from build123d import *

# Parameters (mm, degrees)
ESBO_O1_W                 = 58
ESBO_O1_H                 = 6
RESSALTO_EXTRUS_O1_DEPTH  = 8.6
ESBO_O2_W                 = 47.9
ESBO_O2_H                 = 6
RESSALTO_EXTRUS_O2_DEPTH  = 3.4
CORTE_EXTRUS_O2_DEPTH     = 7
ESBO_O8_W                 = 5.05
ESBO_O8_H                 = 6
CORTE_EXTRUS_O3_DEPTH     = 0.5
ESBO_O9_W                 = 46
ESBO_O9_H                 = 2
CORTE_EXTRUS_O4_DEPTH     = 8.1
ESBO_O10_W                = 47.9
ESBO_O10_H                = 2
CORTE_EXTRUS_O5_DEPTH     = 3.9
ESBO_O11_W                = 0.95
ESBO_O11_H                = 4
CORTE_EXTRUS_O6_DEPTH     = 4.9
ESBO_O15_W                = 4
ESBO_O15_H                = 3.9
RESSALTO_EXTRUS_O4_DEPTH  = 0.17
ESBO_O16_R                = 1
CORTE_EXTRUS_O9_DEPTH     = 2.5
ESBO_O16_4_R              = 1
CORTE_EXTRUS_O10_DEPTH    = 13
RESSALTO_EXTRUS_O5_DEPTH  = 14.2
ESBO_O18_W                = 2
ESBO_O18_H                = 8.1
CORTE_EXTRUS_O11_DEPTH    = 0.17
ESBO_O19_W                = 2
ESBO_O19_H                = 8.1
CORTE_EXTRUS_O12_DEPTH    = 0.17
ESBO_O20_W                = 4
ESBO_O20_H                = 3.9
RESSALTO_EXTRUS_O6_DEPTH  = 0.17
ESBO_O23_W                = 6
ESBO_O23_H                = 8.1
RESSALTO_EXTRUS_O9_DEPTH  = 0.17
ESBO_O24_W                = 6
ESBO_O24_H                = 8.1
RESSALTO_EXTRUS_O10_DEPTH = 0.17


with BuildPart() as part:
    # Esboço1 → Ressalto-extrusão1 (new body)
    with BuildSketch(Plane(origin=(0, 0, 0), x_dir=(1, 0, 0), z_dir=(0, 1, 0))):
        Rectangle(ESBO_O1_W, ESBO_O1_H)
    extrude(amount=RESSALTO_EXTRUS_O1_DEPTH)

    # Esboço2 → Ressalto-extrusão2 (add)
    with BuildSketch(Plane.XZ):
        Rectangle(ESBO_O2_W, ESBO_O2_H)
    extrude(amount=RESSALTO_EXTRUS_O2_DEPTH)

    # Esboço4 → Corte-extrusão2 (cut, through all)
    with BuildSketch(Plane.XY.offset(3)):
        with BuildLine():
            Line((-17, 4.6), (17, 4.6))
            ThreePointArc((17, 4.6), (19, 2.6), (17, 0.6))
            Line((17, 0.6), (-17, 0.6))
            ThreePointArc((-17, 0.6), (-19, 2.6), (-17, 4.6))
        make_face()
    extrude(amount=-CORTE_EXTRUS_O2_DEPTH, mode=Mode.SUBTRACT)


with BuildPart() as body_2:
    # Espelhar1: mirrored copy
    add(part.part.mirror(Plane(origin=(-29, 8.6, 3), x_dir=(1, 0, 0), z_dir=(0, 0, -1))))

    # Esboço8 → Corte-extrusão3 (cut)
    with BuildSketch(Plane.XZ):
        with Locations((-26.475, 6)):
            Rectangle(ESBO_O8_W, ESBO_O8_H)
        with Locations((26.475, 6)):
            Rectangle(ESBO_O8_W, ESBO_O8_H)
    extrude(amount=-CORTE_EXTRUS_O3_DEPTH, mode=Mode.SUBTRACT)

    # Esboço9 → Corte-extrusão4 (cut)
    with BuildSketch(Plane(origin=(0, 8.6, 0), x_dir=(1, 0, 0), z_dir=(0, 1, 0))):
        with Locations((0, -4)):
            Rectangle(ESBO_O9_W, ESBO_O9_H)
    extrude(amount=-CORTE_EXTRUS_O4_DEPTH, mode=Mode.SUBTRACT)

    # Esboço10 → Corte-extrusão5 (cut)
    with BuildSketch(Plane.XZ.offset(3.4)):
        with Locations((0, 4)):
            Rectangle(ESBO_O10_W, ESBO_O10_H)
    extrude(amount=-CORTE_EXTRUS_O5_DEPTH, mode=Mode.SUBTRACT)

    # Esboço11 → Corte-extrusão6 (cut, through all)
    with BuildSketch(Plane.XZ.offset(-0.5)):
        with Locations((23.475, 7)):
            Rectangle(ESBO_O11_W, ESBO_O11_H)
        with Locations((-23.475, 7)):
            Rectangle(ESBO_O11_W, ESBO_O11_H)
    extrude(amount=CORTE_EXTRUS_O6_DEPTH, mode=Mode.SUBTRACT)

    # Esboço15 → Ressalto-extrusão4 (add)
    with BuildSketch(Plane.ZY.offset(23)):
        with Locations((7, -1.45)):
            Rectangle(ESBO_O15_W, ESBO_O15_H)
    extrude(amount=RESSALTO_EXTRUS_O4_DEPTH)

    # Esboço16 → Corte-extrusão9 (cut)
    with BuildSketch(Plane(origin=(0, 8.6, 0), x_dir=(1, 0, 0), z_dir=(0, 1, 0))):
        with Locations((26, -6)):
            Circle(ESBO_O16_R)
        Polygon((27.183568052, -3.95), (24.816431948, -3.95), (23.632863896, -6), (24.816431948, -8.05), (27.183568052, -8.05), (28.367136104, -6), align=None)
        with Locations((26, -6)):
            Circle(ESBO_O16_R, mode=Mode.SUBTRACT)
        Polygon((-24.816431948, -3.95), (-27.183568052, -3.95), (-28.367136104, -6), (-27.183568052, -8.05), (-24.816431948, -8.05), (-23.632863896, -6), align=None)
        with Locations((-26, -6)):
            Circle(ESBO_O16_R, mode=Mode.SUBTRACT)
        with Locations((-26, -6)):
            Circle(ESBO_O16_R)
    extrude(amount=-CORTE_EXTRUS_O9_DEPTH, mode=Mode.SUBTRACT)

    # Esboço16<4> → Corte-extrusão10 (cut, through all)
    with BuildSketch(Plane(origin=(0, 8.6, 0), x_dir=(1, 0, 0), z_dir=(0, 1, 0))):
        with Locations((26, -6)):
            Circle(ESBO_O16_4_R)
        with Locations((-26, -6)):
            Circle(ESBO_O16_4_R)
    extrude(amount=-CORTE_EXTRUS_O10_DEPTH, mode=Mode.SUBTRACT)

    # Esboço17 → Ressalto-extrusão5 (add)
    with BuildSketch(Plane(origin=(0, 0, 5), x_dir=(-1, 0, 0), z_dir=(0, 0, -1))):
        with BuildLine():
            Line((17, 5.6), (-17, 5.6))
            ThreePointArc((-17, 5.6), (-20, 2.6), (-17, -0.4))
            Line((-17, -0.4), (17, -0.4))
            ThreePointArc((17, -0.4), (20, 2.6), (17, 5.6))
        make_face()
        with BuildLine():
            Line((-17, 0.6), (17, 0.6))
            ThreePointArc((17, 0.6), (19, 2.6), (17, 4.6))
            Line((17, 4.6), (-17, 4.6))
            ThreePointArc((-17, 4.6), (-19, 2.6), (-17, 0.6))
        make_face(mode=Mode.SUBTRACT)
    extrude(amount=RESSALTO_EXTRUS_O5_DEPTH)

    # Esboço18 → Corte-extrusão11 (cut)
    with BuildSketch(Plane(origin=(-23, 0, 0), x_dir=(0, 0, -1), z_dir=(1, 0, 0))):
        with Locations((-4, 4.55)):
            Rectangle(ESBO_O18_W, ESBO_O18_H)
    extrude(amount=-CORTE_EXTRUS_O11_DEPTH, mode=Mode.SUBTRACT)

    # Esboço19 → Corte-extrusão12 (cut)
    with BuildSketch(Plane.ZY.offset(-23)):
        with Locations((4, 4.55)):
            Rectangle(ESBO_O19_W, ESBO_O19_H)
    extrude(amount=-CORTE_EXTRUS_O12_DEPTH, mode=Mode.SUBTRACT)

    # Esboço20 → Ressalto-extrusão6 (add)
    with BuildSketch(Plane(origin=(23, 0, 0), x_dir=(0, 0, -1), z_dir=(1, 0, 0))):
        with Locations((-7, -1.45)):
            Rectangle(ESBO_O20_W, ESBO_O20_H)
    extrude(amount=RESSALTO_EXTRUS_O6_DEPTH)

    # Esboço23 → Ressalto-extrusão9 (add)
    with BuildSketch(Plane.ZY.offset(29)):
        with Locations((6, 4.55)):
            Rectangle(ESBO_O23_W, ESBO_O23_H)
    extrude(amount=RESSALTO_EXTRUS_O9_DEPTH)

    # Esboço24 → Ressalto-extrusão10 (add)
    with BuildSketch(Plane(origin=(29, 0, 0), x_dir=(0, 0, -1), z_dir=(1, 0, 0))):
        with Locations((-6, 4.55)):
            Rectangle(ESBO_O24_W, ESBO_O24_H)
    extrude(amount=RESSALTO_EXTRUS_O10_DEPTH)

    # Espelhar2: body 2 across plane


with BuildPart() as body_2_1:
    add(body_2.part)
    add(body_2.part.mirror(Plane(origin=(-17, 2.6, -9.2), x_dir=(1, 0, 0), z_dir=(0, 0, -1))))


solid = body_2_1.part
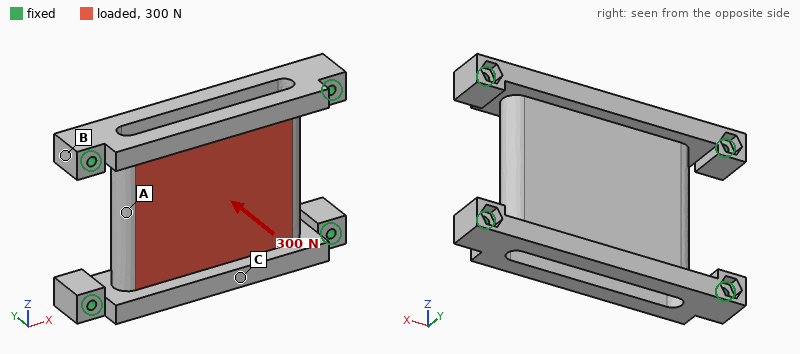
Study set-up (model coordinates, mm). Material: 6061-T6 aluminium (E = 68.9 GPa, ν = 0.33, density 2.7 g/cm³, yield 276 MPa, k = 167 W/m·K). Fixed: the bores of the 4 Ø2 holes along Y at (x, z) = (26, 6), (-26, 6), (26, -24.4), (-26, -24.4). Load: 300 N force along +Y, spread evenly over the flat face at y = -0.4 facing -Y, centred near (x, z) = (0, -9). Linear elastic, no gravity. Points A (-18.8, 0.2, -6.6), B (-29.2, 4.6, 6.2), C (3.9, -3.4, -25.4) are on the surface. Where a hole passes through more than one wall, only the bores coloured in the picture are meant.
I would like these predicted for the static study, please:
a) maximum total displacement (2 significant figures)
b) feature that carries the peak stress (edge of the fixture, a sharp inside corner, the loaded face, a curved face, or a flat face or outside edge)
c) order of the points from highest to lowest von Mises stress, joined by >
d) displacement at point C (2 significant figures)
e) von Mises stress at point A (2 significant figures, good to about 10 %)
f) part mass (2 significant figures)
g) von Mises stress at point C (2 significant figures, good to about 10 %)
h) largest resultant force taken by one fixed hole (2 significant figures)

0.11 mm
a curved face
A > C > B
0.022 mm
51 MPa
18 g
26 MPa
91 N
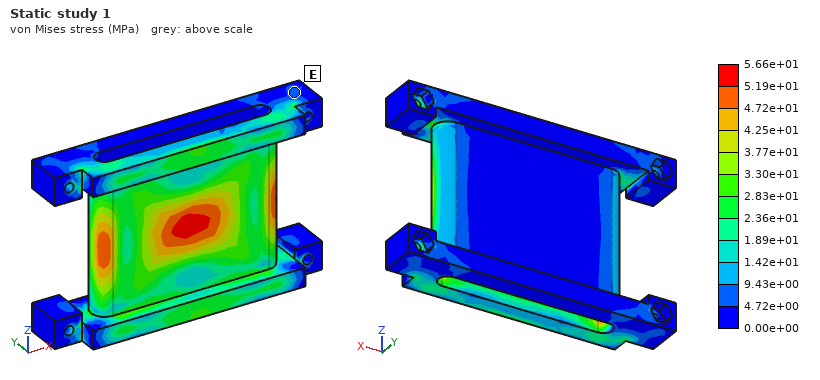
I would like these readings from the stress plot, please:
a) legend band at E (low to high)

4.72e+00 to 9.43e+00 MPa
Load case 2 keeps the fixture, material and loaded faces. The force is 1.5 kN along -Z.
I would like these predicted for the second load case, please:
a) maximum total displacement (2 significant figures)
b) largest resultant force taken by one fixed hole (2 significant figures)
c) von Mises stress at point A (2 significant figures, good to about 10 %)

30 µm
390 N
25 MPa
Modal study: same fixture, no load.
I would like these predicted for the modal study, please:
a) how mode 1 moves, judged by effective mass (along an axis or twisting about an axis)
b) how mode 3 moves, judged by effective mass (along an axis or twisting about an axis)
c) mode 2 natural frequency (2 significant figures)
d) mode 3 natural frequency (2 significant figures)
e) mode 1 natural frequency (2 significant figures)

along Y
twisting about X
6500 Hz
9300 Hz
6100 Hz
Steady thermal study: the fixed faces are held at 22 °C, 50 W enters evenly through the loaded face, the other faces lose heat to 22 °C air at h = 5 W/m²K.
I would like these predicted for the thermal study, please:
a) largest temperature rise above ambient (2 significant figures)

63 K
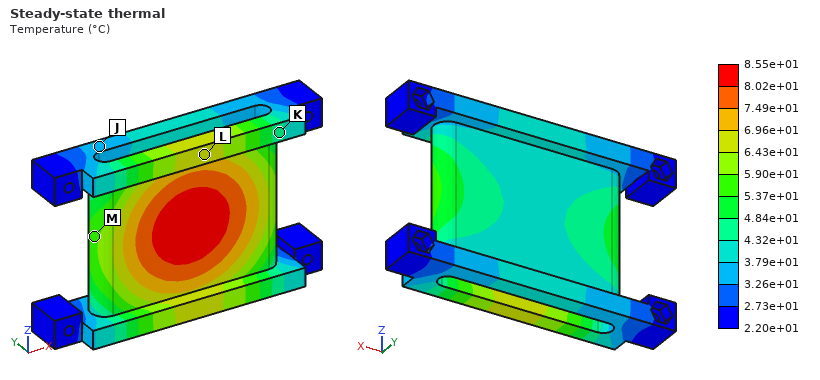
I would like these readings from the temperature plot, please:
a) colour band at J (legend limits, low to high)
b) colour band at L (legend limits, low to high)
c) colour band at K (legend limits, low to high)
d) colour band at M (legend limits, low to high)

3.26e+01 to 3.79e+01 °C
6.43e+01 to 6.96e+01 °C
4.32e+01 to 4.84e+01 °C
5.37e+01 to 5.90e+01 °C
